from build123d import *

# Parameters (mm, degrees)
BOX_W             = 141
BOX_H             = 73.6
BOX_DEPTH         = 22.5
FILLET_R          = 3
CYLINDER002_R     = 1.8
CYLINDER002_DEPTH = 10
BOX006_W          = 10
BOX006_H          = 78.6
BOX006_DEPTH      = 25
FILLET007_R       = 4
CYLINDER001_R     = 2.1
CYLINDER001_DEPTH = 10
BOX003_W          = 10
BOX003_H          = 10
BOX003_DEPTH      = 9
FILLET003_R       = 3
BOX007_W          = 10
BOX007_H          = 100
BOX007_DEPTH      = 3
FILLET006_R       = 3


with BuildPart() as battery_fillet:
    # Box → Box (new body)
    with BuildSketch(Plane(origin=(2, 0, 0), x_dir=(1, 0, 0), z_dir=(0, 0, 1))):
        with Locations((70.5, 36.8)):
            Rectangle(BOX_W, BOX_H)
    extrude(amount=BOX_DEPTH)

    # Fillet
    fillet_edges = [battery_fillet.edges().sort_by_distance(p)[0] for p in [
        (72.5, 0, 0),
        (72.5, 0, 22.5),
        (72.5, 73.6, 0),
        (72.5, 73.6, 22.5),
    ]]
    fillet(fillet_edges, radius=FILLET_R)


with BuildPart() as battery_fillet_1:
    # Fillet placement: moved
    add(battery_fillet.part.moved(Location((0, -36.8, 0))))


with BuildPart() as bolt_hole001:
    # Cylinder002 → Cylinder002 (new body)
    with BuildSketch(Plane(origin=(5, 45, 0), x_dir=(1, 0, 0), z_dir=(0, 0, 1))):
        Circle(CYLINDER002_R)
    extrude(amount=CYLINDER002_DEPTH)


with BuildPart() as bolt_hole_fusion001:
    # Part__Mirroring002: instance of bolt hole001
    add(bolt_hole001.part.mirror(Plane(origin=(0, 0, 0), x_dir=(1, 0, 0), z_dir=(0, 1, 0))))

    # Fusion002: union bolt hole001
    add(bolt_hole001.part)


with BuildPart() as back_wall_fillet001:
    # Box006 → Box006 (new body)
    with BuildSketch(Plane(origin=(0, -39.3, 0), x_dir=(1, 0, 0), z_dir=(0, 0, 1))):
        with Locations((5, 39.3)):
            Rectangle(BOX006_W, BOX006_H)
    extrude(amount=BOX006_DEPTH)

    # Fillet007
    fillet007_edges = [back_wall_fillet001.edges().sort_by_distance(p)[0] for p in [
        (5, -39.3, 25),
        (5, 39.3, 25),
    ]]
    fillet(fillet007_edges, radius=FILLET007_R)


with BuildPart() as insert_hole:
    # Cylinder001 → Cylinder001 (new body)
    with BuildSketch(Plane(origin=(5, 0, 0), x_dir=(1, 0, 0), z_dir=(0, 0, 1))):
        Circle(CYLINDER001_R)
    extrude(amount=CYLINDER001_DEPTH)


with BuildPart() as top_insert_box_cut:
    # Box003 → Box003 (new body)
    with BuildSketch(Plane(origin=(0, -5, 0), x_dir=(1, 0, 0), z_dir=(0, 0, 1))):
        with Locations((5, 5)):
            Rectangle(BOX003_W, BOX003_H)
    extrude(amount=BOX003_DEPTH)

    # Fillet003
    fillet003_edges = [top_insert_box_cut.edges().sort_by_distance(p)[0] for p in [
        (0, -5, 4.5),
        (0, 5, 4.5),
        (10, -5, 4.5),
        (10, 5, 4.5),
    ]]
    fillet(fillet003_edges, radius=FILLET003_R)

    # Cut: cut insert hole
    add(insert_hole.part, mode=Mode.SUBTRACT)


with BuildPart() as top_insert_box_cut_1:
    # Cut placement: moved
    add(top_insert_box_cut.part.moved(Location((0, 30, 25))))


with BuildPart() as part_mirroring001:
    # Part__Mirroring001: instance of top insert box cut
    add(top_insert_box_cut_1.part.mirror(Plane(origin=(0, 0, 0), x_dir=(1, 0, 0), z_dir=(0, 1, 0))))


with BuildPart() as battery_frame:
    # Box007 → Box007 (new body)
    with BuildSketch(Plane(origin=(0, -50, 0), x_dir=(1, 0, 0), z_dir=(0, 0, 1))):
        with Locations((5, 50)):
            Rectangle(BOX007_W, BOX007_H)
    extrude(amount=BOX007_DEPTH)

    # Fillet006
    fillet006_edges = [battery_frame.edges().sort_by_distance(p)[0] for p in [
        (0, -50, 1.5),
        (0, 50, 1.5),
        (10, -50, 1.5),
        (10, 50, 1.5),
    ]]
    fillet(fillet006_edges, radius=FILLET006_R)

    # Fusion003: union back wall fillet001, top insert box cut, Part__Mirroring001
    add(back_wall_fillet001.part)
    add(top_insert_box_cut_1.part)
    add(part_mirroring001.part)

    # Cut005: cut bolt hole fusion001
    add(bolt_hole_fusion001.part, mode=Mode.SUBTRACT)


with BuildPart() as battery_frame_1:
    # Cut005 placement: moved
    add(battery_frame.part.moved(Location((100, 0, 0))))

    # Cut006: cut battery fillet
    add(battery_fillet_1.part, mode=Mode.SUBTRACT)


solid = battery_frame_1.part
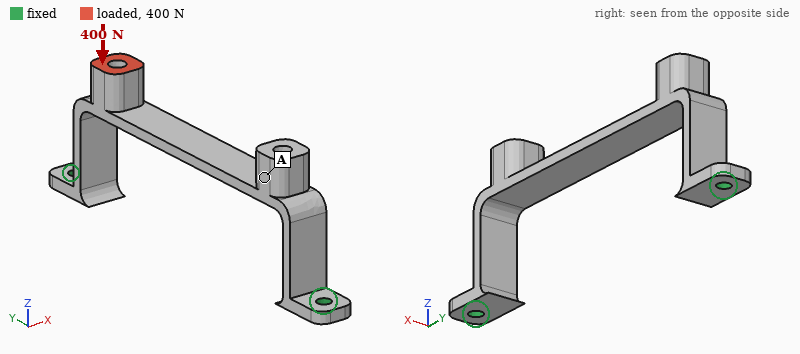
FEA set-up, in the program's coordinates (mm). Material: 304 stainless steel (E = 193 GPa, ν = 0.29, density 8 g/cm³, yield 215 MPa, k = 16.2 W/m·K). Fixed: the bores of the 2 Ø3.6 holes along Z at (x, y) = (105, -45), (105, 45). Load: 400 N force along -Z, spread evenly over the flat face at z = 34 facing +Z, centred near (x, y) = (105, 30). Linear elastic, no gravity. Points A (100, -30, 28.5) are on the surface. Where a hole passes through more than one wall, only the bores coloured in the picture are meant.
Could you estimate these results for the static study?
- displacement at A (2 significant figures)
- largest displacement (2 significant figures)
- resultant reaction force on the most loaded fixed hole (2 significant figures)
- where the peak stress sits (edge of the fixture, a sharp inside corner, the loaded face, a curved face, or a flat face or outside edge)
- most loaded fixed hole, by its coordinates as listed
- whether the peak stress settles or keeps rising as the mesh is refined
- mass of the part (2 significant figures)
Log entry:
0.037 mm
0.12 mm
370 N
edge of the fixture
(105, 45)
keeps rising
41 g
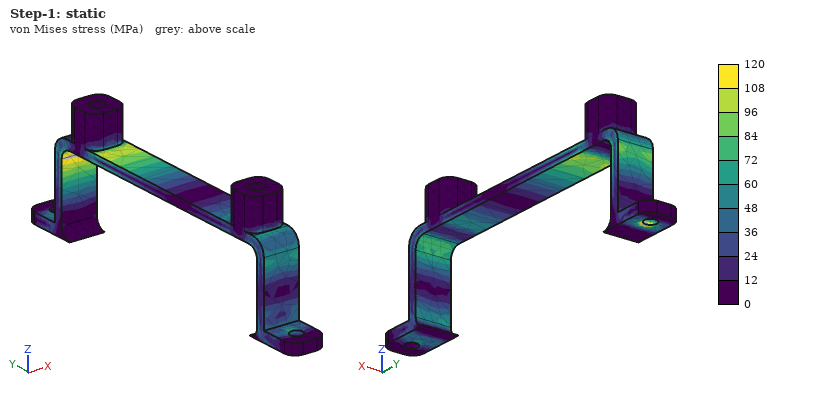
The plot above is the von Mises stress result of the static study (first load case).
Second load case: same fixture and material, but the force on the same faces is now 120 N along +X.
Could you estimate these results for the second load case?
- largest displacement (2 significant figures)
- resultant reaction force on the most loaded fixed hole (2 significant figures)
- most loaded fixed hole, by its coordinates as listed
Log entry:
0.12 mm
110 N
(105, 45)
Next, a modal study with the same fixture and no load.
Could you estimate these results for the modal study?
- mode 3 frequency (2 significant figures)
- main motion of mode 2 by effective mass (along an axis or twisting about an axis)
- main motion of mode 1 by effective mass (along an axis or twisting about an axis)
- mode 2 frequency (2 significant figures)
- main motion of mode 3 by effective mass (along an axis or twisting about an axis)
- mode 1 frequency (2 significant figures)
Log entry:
1900 Hz
along X
along Y
1600 Hz
along Z
1400 Hz
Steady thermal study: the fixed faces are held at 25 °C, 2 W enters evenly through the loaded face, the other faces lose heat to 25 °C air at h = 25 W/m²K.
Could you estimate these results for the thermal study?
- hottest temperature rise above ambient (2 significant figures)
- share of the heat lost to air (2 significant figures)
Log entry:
52 K
76 %
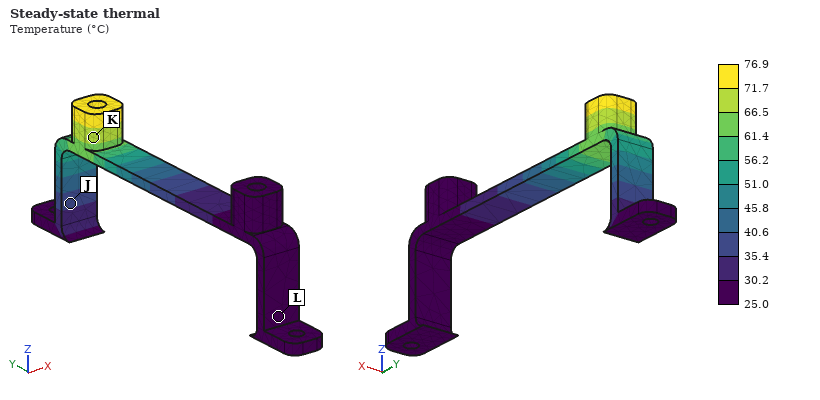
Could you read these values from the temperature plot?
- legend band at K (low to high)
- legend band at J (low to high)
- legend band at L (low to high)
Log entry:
66.5 to 71.7 °C
35.4 to 40.6 °C
25.0 to 30.2 °C
